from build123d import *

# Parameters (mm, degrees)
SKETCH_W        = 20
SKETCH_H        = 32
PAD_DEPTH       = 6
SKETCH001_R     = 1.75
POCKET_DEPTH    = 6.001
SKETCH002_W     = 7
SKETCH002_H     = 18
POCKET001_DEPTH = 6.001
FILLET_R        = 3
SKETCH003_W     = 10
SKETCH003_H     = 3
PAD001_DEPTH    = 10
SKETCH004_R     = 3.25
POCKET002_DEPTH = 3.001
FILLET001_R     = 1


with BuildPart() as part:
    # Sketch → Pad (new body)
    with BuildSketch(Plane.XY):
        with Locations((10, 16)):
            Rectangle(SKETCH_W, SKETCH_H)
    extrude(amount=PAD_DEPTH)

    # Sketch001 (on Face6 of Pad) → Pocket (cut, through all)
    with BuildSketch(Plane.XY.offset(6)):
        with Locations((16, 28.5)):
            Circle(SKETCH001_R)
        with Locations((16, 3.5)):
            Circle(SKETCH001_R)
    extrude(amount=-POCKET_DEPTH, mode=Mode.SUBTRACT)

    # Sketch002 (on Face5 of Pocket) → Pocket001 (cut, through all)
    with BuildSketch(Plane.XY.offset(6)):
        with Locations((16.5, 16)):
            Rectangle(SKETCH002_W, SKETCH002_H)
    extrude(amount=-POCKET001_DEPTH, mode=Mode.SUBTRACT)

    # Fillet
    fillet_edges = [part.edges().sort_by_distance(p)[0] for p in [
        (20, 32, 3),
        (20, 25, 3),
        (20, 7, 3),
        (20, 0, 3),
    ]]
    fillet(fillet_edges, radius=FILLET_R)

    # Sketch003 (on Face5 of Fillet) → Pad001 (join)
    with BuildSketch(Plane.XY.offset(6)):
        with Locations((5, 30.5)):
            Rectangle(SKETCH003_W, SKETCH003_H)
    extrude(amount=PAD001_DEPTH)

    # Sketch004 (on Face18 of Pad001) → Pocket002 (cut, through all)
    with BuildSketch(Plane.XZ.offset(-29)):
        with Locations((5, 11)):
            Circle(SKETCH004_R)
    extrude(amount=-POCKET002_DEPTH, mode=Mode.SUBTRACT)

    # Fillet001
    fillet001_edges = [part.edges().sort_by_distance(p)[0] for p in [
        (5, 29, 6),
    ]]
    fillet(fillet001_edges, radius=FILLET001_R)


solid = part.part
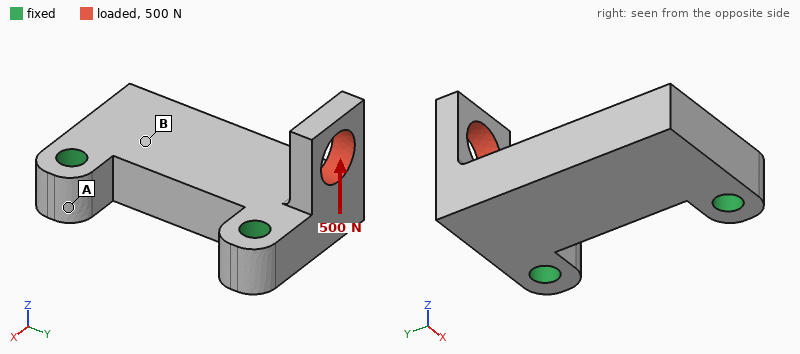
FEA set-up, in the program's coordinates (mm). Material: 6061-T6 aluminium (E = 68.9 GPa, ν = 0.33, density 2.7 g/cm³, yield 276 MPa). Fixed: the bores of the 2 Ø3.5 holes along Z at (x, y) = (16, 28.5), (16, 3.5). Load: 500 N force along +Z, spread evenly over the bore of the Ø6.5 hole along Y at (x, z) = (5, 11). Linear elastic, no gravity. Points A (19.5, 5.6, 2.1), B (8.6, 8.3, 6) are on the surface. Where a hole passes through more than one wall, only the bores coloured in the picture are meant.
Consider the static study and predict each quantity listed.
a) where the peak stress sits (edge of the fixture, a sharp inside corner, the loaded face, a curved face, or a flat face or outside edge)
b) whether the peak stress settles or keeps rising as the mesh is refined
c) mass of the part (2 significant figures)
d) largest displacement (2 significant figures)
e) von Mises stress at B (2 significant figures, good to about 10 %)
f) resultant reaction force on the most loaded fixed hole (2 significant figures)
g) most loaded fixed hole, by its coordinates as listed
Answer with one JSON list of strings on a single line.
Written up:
["edge of the fixture", "keeps rising", "8.4 g", "47 µm", "17 MPa", "510 N", "(16, 28.5)"]
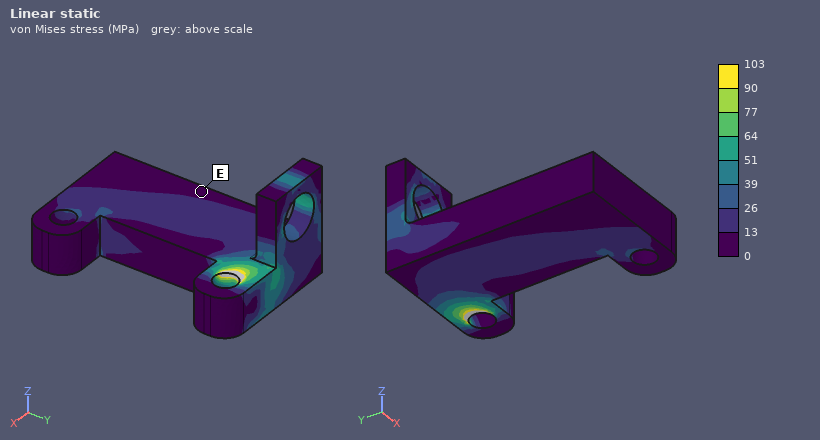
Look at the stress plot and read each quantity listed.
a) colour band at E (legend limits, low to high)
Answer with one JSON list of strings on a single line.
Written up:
["0 to 13 MPa"]
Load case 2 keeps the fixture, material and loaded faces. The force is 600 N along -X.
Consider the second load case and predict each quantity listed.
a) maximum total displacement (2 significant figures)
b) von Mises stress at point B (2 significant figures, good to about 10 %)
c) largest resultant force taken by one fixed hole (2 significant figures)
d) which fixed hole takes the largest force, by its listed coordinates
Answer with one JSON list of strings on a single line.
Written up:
["96 µm", "21 MPa", "640 N", "(16, 28.5)"]
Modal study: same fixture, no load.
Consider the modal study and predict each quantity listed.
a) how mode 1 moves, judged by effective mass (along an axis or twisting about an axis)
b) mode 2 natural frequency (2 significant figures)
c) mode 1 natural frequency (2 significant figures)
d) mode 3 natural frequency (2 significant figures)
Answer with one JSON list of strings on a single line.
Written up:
["along Z", "15 kHz", "12 kHz", "21 kHz"]
